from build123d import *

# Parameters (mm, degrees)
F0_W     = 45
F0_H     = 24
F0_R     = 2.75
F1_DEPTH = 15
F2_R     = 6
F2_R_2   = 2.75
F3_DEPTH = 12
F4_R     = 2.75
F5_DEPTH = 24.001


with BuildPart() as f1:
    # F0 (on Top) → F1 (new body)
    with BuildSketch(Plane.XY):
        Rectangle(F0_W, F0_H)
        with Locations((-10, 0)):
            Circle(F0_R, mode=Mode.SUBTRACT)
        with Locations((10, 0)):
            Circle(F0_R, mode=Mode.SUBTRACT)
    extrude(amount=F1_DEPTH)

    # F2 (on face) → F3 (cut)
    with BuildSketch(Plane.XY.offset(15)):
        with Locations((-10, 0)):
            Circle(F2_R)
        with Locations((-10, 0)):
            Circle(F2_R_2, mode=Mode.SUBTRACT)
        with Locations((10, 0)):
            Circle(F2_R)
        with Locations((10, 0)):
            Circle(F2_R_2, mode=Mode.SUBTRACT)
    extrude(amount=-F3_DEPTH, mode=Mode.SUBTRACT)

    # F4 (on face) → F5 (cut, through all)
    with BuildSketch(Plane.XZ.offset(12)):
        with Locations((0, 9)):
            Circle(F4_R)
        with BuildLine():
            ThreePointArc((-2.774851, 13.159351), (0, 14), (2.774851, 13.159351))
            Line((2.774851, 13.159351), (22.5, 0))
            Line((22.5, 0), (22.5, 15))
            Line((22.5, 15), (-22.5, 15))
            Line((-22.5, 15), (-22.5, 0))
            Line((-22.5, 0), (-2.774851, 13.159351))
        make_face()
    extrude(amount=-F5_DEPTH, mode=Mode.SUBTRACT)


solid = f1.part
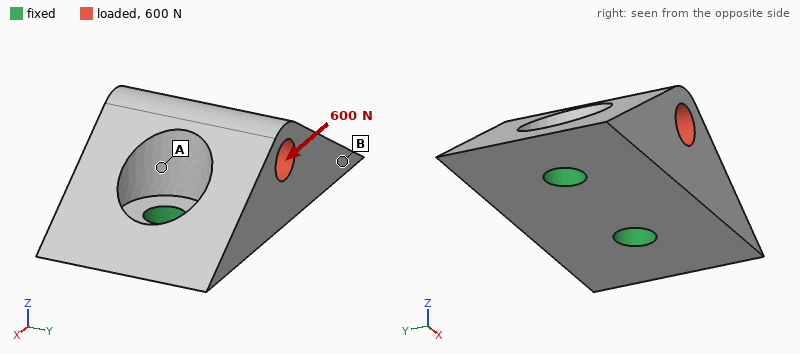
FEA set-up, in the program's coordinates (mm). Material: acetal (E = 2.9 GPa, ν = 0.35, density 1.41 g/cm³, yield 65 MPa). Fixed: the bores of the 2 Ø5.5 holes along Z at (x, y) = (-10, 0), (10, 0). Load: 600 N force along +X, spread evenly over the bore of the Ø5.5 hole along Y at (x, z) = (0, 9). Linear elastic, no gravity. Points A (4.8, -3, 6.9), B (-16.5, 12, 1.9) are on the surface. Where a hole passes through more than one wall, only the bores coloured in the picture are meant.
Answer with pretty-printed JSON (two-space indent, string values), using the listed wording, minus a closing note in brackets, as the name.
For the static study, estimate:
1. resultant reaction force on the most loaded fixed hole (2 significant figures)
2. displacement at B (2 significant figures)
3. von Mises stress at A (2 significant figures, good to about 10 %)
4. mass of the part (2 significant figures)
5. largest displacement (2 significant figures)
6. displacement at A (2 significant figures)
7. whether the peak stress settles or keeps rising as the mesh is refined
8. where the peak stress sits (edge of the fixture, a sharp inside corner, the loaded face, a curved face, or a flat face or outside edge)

{
  "resultant reaction force on the most loaded fixed hole": "370 N",
  "displacement at B": "62 µm",
  "von Mises stress at A": "5.4 MPa",
  "mass of the part": "8.7 g",
  "largest displacement": "81 µm",
  "displacement at A": "40 µm",
  "whether the peak stress settles or keeps rising as the mesh is refined": "keeps rising",
  "where the peak stress sits": "edge of the fixture"
}
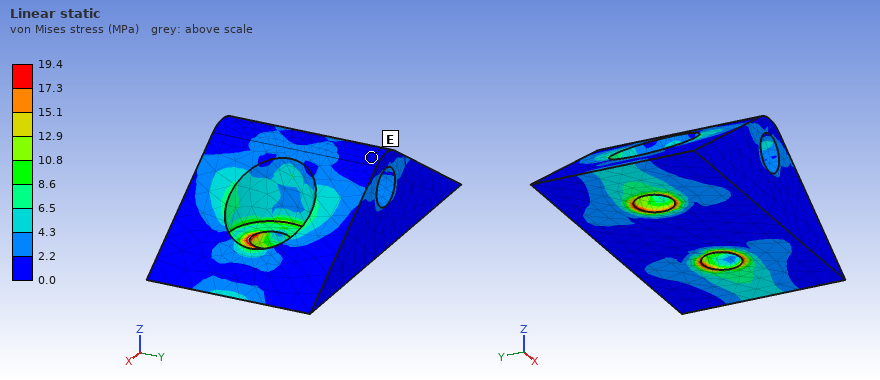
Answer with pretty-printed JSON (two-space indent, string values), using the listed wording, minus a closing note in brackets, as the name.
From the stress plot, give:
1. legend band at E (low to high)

{
  "legend band at E": "0.0 to 2.2 MPa"
}
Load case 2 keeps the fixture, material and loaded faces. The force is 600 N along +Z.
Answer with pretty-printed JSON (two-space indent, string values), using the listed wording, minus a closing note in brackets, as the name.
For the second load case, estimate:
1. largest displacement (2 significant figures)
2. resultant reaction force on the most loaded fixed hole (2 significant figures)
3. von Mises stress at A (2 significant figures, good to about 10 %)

{
  "largest displacement": "63 µm",
  "resultant reaction force on the most loaded fixed hole": "320 N",
  "von Mises stress at A": "5.5 MPa"
}
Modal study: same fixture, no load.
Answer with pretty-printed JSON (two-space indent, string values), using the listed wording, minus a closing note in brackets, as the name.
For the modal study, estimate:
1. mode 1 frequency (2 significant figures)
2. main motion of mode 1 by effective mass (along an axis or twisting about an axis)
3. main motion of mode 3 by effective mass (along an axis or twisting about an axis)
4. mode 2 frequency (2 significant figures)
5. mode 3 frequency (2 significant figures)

{
  "mode 1 frequency": "3100 Hz",
  "main motion of mode 1 by effective mass": "along Y",
  "main motion of mode 3 by effective mass": "along Z",
  "mode 2 frequency": "6400 Hz",
  "mode 3 frequency": "6700 Hz"
}
